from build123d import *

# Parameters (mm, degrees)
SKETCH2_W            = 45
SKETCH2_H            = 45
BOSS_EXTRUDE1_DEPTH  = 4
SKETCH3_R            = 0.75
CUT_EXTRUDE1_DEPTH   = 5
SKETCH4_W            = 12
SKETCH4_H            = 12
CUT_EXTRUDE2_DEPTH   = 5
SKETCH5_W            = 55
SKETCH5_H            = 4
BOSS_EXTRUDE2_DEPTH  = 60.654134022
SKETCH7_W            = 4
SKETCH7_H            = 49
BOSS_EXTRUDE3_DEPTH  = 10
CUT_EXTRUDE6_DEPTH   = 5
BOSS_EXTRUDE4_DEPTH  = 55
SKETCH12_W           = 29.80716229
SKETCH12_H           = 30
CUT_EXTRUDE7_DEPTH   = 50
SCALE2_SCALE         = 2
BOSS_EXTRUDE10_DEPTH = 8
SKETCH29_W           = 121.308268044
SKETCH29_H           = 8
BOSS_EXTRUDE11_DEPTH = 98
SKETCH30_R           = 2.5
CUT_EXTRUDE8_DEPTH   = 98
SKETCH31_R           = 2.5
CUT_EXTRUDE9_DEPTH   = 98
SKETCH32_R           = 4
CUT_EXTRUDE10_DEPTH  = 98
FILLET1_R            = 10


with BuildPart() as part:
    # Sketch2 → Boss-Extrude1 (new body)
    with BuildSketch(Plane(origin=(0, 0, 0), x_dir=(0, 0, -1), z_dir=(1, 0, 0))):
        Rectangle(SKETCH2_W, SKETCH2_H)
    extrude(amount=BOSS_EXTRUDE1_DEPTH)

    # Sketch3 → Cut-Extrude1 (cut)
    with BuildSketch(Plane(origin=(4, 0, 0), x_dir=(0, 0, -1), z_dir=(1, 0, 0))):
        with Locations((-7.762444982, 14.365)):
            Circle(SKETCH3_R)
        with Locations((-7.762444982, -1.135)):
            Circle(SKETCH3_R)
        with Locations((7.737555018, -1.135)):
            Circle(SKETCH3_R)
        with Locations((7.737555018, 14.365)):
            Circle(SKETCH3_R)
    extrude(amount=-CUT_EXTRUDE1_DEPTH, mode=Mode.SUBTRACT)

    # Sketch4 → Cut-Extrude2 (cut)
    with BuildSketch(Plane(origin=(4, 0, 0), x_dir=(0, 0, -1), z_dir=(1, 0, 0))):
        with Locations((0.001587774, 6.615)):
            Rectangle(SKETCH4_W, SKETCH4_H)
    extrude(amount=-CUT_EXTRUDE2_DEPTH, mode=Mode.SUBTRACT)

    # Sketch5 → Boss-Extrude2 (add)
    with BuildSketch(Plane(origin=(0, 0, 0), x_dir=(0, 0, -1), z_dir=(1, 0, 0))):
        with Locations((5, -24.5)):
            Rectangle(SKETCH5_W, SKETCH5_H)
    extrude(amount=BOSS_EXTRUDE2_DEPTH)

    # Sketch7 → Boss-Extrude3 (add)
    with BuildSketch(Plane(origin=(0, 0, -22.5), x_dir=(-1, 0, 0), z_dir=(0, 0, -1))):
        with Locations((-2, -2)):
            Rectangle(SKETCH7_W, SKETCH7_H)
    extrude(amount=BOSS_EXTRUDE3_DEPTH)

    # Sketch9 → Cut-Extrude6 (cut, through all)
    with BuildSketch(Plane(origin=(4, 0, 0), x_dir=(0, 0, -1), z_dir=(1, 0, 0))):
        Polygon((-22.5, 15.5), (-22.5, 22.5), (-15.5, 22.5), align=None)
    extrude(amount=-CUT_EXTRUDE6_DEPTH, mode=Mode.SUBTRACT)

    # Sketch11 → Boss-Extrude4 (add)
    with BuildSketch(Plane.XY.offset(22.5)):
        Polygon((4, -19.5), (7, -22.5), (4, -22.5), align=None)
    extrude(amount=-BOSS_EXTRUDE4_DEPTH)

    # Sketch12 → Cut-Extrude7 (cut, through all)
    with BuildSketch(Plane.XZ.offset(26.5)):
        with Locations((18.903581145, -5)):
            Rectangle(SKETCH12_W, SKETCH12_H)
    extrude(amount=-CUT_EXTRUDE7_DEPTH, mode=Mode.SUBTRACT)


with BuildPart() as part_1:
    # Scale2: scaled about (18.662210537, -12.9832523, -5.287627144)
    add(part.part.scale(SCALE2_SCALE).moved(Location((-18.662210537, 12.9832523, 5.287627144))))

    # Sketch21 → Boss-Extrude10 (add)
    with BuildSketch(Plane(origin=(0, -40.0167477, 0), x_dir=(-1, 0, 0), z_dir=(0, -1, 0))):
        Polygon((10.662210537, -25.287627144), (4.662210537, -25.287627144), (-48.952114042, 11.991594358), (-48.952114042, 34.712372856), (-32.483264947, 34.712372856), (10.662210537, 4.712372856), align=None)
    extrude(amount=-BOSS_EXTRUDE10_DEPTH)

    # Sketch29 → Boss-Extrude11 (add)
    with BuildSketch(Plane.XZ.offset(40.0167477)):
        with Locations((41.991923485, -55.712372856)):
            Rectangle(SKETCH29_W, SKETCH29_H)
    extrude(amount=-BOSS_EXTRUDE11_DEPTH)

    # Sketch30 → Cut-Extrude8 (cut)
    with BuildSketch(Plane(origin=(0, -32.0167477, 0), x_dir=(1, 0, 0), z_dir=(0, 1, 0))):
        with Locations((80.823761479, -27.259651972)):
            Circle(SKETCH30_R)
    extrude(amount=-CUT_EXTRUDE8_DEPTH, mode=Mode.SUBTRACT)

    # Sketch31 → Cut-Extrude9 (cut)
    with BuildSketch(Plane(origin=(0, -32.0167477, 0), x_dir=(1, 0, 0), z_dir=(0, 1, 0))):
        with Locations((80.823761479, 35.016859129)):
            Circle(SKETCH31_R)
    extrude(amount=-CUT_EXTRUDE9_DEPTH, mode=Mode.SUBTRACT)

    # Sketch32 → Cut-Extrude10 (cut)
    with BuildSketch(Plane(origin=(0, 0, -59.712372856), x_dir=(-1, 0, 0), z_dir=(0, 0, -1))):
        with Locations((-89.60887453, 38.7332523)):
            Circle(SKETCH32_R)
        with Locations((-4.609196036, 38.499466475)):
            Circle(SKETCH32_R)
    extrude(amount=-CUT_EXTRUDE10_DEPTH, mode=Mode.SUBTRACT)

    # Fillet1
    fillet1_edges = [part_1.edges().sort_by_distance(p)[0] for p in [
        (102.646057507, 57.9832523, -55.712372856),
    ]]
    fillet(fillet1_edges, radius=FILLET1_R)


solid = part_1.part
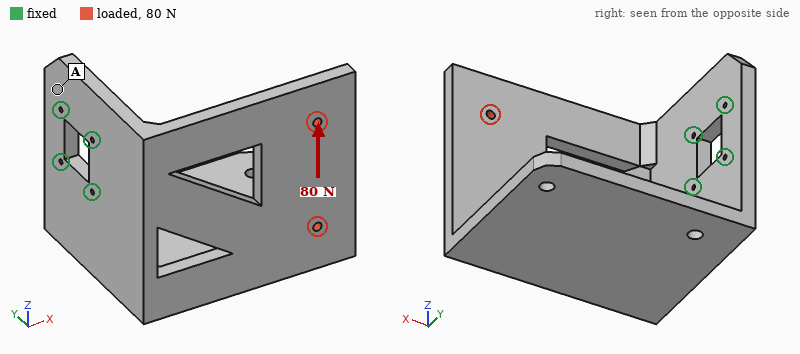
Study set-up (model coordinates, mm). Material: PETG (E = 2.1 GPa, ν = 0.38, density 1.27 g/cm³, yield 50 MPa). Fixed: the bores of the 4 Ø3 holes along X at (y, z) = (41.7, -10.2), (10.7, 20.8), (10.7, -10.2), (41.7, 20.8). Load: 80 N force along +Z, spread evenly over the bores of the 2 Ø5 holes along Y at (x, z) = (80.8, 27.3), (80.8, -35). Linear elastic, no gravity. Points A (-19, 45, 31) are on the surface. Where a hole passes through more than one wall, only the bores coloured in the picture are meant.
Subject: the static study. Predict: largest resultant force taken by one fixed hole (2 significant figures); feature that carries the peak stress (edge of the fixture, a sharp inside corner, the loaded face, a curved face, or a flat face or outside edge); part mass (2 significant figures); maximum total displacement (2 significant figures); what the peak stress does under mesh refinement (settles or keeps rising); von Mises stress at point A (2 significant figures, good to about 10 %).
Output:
200 N
edge of the fixture
320 g
2.0 mm
keeps rising
0.79 MPa
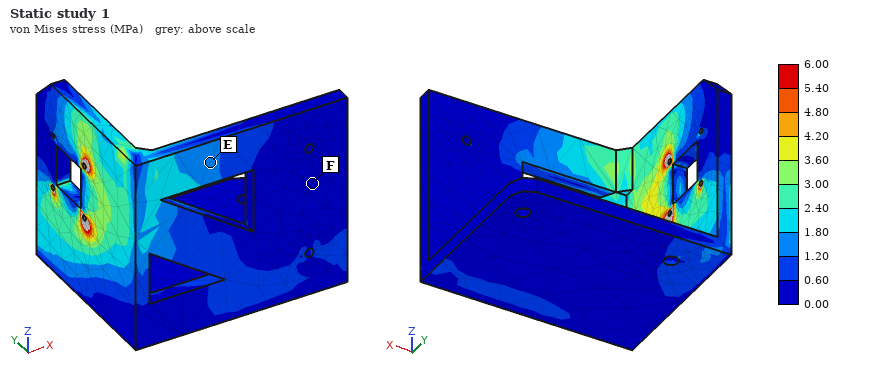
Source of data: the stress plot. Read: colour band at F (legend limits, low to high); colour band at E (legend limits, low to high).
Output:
0.00 to 0.60 MPa
1.20 to 1.80 MPa
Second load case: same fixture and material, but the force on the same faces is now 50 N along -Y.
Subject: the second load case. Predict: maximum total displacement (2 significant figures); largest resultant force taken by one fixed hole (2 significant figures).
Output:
2.2 mm
110 N
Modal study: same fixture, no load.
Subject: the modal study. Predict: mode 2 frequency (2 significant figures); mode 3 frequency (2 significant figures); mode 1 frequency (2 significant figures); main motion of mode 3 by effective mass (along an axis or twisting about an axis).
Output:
100 Hz
250 Hz
87 Hz
twisting about X
